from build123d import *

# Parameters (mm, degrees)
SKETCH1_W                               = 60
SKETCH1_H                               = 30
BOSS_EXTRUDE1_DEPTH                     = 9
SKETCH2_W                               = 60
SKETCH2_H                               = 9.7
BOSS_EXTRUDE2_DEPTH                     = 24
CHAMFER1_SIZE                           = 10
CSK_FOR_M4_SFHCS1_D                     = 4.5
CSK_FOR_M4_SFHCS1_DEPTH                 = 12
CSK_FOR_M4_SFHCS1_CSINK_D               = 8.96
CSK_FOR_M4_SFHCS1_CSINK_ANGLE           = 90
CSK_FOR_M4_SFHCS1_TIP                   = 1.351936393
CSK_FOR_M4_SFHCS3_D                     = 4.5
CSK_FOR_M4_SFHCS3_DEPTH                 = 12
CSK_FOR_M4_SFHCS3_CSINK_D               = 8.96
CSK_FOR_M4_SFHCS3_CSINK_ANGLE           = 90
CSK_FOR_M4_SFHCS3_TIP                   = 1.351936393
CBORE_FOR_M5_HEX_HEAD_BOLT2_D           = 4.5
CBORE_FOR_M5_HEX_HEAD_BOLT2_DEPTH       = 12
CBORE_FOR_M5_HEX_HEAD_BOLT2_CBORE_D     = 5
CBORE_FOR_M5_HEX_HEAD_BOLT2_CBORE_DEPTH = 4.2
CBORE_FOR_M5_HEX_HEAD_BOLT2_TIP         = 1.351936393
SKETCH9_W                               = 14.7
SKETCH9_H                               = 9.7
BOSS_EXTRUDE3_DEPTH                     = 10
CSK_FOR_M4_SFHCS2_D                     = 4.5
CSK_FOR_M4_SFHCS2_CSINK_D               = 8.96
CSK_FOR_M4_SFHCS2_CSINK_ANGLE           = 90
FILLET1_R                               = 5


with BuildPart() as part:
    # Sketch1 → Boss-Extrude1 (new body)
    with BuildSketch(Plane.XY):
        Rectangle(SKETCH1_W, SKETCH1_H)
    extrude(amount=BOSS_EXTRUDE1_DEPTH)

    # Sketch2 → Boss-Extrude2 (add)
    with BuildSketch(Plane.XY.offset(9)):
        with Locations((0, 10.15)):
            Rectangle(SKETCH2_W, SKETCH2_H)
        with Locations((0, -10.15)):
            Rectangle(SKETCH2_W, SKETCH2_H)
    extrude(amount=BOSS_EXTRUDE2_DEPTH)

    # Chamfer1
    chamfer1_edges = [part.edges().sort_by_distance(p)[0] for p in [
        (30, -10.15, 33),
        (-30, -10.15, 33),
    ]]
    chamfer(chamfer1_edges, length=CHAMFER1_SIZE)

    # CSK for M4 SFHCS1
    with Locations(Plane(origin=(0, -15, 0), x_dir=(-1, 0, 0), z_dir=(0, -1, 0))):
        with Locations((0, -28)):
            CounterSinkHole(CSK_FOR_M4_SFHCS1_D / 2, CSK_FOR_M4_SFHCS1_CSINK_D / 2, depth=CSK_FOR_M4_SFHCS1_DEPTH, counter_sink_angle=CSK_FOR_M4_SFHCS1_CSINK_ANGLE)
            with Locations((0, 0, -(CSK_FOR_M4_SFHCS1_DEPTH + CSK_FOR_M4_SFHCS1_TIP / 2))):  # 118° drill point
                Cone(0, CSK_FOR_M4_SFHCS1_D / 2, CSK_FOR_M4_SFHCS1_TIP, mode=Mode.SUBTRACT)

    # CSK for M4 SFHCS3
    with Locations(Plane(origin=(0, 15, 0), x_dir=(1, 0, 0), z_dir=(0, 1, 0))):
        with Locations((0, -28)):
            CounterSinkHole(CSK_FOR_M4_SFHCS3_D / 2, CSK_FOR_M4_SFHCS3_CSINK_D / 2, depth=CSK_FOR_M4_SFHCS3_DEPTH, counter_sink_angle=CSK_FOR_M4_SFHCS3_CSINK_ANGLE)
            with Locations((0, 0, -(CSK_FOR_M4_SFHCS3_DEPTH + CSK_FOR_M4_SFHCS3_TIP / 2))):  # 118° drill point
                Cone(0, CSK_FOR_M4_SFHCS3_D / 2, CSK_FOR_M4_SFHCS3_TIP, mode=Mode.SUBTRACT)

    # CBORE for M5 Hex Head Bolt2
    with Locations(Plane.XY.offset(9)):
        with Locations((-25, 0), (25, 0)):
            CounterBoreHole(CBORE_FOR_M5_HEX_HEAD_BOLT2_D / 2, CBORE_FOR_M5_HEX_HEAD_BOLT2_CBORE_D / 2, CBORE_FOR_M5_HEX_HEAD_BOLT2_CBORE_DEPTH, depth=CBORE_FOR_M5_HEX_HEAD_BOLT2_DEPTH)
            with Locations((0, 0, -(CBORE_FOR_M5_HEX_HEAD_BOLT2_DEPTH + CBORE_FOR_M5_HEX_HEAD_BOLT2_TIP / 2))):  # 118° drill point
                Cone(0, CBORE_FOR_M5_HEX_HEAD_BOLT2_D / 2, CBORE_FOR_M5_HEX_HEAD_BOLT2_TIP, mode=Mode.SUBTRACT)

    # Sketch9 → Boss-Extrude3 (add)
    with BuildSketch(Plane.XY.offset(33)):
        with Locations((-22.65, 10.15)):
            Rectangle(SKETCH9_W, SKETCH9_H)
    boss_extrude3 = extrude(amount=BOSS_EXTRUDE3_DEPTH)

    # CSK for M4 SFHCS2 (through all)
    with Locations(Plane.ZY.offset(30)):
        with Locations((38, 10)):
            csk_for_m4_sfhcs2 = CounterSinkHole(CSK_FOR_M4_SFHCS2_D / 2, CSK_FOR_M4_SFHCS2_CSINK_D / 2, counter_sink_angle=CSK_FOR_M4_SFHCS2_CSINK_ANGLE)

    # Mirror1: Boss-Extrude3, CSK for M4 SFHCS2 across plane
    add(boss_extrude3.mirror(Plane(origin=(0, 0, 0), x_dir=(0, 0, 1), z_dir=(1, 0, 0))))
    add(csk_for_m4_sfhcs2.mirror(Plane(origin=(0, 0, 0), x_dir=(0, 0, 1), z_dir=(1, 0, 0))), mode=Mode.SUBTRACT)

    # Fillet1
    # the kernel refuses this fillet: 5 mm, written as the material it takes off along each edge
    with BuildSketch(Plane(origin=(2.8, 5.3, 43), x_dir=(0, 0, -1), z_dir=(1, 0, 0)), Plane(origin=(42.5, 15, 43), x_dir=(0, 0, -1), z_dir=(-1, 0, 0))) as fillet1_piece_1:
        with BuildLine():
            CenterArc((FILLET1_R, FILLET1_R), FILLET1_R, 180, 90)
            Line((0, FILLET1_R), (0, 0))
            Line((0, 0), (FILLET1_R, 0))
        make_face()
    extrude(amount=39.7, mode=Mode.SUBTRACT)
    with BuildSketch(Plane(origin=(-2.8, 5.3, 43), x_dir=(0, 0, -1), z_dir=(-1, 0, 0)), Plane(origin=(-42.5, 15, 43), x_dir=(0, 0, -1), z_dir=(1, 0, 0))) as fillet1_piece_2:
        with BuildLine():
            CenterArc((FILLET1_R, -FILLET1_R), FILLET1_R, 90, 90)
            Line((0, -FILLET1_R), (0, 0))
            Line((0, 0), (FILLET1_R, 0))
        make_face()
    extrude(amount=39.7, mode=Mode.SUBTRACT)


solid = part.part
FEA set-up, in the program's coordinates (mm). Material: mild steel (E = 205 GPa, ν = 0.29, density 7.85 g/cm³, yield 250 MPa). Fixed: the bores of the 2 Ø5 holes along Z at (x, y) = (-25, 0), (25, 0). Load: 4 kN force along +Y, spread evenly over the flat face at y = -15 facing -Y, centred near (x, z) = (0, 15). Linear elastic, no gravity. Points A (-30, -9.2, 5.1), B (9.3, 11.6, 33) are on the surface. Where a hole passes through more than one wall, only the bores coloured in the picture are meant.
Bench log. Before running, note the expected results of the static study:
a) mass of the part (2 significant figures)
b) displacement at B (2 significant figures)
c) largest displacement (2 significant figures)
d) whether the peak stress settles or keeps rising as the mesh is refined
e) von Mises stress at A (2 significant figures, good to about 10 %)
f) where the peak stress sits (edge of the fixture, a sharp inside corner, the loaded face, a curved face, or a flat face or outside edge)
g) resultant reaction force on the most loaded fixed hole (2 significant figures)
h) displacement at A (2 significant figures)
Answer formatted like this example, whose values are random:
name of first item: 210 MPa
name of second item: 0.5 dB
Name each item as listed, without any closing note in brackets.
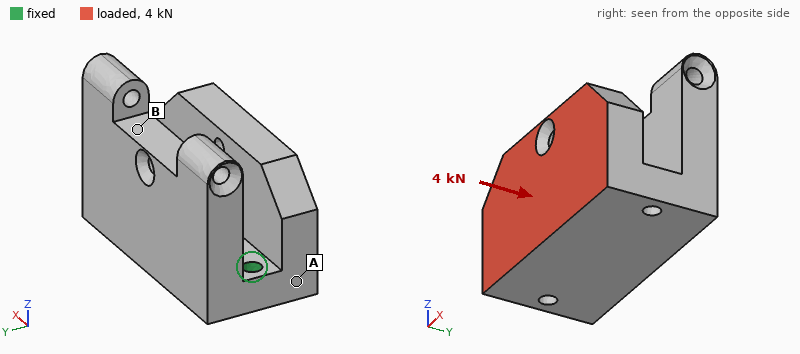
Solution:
mass of the part: 350 g
displacement at B: 22 µm
largest displacement: 45 µm
whether the peak stress settles or keeps rising as the mesh is refined: keeps rising
von Mises stress at A: 34 MPa
where the peak stress sits: edge of the fixture
resultant reaction force on the most loaded fixed hole: 2.0 kN
displacement at A: 7.7 µm
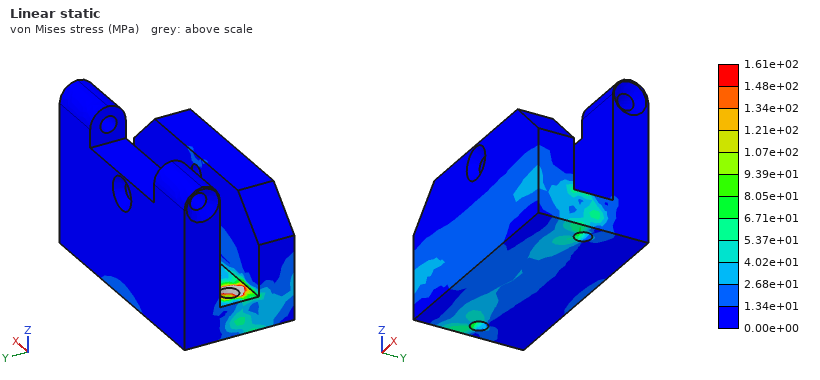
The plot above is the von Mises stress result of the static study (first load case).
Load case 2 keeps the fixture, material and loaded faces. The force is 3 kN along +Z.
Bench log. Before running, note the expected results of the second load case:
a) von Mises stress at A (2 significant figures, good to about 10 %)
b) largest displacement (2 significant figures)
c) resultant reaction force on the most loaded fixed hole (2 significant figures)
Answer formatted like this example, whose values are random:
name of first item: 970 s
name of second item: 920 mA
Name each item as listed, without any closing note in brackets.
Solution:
von Mises stress at A: 29 MPa
largest displacement: 42 µm
resultant reaction force on the most loaded fixed hole: 1.5 kN
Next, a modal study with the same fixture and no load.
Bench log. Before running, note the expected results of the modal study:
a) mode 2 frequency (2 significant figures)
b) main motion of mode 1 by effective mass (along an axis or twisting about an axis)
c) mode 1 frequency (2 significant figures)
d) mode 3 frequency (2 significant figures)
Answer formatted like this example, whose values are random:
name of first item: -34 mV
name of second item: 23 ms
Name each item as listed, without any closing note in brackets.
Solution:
mode 2 frequency: 6000 Hz
main motion of mode 1 by effective mass: along Y
mode 1 frequency: 3000 Hz
mode 3 frequency: 7300 Hz
